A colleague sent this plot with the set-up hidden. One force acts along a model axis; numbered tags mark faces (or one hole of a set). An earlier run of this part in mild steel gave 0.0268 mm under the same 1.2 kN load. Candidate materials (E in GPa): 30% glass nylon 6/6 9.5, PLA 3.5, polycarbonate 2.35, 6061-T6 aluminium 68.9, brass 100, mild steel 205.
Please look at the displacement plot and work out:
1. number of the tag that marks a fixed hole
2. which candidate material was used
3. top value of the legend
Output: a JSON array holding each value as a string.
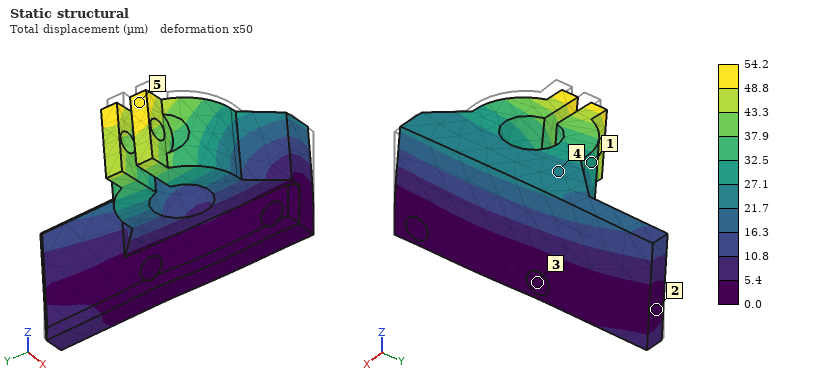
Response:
["3", "brass", "54.2 µm"]
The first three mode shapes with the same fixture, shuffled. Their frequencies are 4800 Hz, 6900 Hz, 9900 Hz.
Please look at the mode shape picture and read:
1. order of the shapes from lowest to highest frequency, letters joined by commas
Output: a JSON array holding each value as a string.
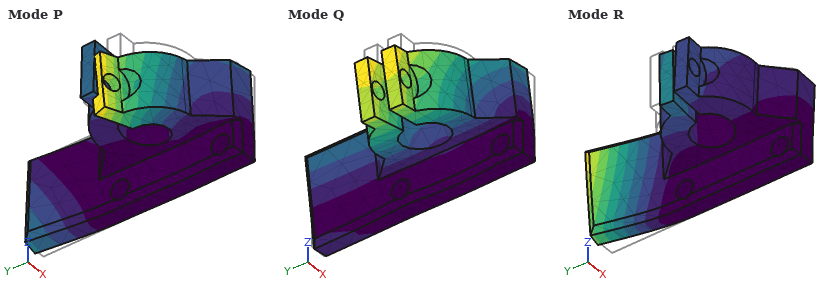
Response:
["Q, R, P"]
